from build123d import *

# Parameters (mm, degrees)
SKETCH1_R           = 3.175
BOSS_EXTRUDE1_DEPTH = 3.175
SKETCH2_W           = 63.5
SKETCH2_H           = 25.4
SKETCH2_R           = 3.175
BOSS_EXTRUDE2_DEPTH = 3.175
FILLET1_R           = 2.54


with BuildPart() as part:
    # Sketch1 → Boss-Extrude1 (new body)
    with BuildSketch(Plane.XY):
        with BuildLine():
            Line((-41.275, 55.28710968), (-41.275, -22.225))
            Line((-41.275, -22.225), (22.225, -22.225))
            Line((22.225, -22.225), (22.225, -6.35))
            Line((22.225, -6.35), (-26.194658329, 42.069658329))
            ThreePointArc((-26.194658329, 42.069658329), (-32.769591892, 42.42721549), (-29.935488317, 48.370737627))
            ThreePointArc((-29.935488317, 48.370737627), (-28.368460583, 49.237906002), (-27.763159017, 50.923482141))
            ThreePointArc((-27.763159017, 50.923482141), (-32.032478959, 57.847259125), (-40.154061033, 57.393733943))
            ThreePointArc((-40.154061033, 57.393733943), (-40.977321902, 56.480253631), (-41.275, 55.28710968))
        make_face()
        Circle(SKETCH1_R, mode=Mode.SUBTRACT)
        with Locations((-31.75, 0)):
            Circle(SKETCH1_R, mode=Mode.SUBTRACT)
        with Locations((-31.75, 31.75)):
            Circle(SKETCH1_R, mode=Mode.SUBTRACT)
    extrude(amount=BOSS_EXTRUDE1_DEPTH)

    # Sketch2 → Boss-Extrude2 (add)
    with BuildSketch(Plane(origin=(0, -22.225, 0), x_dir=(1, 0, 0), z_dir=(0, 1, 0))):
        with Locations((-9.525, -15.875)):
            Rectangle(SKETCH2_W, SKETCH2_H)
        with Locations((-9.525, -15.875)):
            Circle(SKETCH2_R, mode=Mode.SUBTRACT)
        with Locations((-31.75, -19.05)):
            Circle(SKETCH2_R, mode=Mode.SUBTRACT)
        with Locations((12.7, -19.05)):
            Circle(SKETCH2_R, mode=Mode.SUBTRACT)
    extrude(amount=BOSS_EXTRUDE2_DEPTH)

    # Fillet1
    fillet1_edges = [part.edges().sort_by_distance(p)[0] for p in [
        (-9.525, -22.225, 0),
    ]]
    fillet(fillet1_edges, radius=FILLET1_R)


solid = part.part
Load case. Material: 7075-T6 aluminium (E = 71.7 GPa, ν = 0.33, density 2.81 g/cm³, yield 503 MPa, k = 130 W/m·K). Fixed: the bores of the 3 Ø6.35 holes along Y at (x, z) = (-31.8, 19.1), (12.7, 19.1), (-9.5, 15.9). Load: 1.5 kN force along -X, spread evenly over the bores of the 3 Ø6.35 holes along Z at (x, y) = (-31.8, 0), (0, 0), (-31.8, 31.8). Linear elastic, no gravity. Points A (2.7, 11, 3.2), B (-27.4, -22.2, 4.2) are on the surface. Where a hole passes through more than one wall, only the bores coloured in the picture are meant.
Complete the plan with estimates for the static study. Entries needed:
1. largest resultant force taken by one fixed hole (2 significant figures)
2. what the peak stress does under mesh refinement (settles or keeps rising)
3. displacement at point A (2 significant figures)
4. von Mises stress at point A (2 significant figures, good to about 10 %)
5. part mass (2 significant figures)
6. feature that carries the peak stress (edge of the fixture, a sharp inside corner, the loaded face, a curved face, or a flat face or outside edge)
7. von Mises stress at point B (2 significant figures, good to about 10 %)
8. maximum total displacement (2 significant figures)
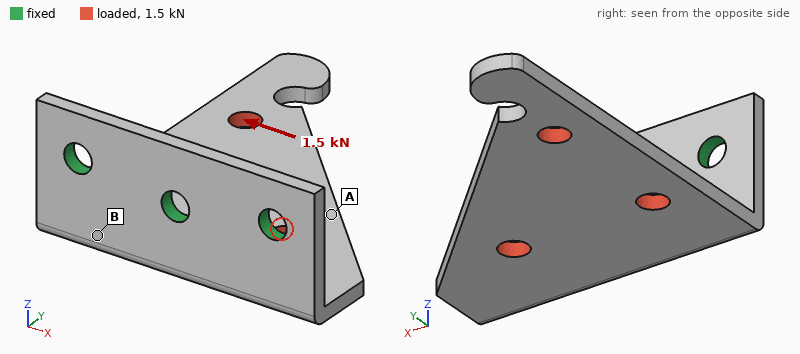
1.1 kN
keeps rising
0.30 mm
40 MPa
40 g
edge of the fixture
89 MPa
0.78 mm
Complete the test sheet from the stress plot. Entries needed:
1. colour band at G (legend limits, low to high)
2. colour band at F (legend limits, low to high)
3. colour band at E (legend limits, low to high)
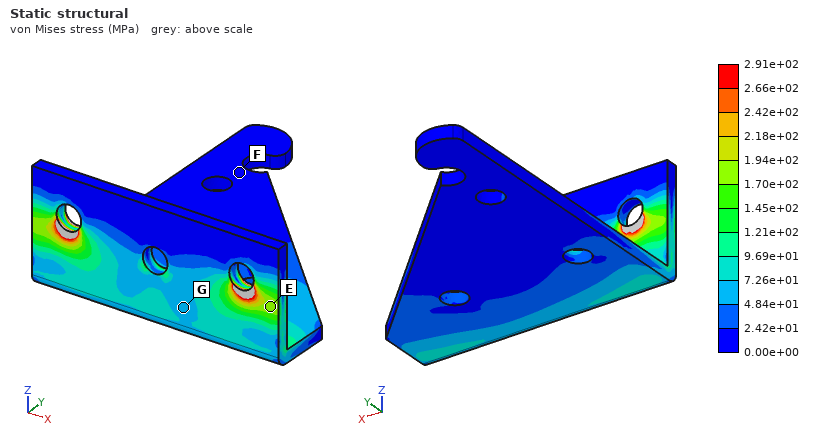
4.84e+01 to 7.26e+01 MPa
0.00e+00 to 2.42e+01 MPa
1.70e+02 to 1.94e+02 MPa
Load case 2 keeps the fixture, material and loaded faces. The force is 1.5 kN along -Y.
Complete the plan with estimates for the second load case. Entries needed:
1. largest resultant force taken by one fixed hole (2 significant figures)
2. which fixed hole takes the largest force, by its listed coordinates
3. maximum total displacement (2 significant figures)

900 N
(-9.5, 15.9)
1.1 mm
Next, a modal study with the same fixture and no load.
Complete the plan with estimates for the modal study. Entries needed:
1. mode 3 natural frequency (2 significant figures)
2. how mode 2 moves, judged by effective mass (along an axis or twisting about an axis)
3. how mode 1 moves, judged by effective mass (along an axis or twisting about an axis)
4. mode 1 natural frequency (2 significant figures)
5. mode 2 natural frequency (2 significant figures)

2100 Hz
along X
along Z
550 Hz
1900 Hz
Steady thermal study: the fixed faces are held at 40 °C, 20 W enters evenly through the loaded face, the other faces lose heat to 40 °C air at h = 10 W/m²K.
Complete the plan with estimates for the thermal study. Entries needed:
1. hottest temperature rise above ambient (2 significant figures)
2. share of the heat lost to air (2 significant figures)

46 K
9.4 %
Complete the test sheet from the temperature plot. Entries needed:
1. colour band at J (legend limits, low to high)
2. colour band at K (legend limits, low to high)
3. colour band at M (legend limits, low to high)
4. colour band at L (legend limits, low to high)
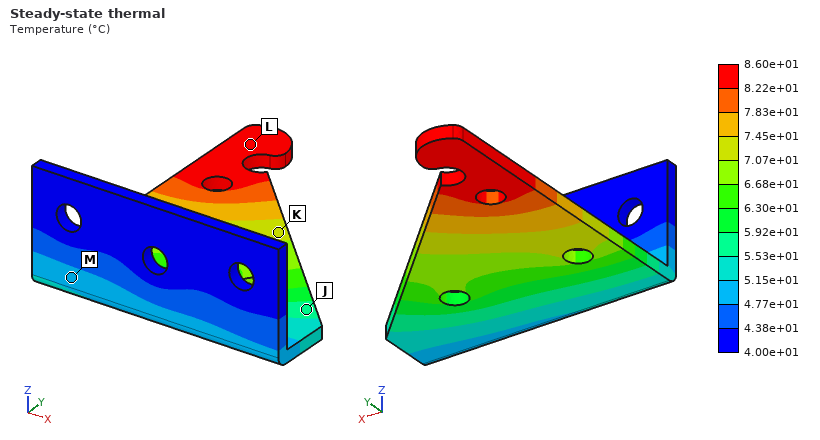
5.53e+01 to 5.92e+01 °C
7.07e+01 to 7.45e+01 °C
4.77e+01 to 5.15e+01 °C
8.22e+01 to 8.60e+01 °C
